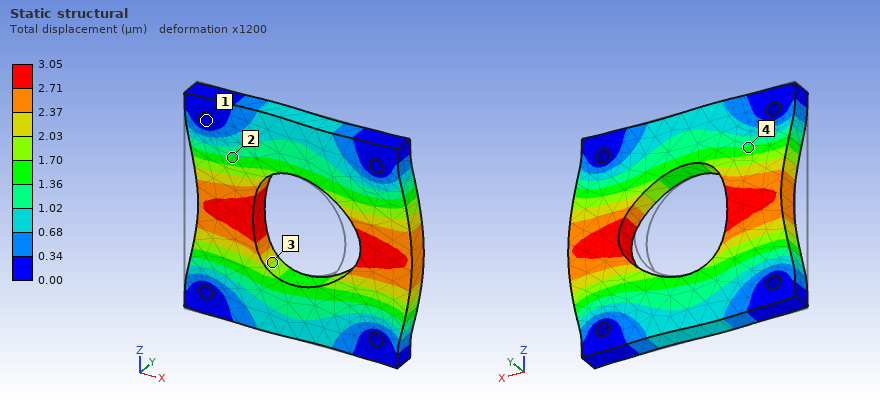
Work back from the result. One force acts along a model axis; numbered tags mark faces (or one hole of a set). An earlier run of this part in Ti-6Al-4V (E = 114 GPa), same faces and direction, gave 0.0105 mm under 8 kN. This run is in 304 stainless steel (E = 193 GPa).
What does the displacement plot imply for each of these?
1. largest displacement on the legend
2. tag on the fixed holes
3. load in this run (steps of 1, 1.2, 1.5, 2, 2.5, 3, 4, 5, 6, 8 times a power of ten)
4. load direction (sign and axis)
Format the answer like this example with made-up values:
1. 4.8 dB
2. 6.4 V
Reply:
1. 3.05 µm
2. 1
3. 4 kN
4. +X
